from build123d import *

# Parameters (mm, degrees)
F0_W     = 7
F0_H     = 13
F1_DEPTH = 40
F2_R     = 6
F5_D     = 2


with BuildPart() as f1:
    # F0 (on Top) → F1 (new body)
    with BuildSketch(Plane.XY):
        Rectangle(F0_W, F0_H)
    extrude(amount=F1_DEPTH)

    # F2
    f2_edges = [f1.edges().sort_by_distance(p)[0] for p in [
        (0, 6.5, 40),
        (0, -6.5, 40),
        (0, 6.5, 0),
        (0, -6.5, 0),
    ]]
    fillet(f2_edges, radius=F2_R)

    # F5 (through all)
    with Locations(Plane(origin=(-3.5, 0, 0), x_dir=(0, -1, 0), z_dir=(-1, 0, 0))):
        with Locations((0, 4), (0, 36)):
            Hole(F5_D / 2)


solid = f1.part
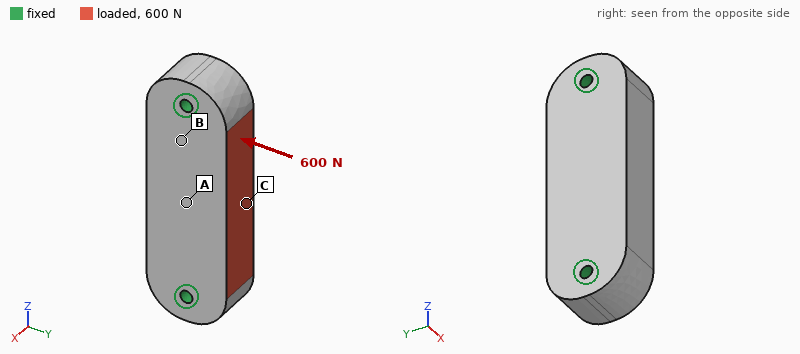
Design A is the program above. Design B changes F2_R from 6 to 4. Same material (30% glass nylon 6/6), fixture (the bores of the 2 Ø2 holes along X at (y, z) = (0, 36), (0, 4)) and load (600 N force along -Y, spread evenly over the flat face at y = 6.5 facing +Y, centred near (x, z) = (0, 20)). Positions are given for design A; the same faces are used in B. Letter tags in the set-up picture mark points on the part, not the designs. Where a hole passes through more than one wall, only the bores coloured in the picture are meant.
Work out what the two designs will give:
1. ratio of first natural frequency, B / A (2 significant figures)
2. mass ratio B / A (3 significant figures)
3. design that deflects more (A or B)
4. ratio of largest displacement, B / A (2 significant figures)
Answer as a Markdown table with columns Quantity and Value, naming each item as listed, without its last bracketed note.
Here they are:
| Quantity | Value |
|---|---|
| ratio of first natural frequency, B / A | 1.0 |
| mass ratio B / A | 1.04 |
| design that deflects more | A |
| ratio of largest displacement, B / A | 0.89 |
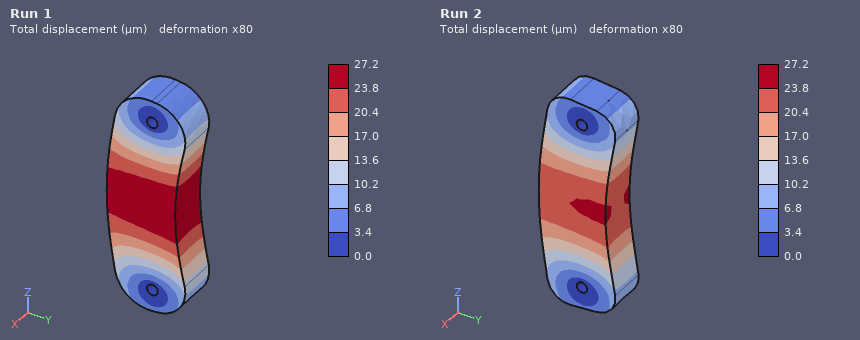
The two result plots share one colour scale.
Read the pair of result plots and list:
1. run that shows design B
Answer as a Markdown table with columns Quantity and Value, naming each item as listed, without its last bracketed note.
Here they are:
| Quantity | Value |
|---|---|
| run that shows design B | Run 2 |
